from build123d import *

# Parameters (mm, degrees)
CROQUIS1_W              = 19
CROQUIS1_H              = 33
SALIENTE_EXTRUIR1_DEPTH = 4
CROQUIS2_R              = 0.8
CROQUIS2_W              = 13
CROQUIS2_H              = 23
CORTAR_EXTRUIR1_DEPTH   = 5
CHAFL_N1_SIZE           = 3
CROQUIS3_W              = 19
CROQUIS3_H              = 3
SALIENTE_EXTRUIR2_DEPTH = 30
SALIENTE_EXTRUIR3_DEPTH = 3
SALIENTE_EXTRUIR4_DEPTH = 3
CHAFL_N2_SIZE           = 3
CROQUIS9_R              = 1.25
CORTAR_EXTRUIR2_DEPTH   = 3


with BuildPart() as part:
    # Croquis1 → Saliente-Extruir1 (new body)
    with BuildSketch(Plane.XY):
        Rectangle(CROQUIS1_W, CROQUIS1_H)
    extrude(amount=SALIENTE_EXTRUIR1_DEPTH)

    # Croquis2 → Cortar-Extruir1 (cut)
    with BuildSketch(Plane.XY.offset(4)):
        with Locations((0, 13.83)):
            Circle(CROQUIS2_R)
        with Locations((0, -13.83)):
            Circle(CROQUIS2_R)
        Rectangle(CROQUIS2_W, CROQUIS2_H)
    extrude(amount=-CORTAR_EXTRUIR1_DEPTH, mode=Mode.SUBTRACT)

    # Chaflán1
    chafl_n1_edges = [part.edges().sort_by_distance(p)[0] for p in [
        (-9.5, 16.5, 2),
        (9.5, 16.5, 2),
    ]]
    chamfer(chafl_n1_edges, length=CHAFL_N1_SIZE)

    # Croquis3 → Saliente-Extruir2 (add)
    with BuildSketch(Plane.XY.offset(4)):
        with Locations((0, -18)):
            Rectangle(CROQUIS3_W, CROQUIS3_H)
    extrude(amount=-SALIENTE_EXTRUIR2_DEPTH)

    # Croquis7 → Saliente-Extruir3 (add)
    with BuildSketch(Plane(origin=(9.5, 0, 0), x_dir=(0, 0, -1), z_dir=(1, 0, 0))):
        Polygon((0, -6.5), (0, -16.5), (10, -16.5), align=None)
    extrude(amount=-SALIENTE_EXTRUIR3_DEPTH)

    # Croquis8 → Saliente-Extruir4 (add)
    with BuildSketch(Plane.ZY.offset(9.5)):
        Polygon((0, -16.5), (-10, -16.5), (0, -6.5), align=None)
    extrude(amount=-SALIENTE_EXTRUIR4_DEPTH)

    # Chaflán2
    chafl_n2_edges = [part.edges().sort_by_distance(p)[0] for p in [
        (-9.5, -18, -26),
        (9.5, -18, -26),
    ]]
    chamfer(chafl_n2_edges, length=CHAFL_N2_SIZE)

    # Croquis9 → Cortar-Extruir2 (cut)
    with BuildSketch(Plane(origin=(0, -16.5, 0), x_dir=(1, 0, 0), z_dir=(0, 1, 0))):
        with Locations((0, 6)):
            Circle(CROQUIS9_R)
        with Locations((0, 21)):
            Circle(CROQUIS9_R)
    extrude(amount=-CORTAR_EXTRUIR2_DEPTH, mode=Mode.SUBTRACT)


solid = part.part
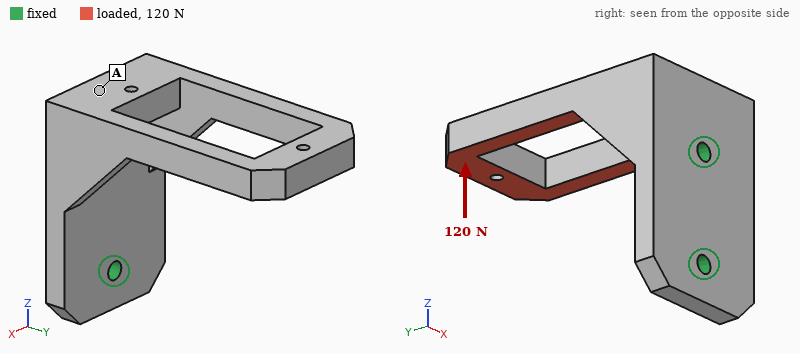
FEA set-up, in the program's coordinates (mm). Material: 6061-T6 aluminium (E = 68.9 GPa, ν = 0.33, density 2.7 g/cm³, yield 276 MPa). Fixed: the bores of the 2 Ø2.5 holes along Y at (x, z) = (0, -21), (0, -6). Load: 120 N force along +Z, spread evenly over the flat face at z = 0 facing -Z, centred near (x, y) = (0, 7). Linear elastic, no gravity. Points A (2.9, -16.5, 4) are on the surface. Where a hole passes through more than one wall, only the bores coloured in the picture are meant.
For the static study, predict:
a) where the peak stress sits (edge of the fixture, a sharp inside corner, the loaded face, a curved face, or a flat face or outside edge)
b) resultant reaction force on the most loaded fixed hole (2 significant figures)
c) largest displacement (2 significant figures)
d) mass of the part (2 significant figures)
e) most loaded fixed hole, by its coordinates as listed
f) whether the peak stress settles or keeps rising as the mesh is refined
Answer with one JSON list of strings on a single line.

["edge of the fixture", "150 N", "0.27 mm", "8.7 g", "(0, -21)", "keeps rising"]
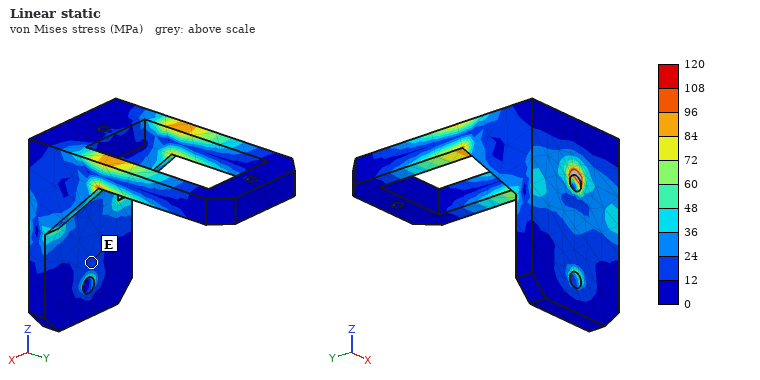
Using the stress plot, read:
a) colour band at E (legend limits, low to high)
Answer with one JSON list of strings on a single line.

["12 to 24 MPa"]
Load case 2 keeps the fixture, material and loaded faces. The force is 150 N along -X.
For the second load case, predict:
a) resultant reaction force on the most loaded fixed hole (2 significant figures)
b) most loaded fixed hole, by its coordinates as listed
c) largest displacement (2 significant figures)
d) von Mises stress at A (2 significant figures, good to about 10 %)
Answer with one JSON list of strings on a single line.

["200 N", "(0, -6)", "0.32 mm", "30 MPa"]
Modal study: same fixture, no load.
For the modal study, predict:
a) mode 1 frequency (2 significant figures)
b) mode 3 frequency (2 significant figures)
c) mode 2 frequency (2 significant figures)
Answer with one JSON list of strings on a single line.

["2600 Hz", "7400 Hz", "2700 Hz"]
